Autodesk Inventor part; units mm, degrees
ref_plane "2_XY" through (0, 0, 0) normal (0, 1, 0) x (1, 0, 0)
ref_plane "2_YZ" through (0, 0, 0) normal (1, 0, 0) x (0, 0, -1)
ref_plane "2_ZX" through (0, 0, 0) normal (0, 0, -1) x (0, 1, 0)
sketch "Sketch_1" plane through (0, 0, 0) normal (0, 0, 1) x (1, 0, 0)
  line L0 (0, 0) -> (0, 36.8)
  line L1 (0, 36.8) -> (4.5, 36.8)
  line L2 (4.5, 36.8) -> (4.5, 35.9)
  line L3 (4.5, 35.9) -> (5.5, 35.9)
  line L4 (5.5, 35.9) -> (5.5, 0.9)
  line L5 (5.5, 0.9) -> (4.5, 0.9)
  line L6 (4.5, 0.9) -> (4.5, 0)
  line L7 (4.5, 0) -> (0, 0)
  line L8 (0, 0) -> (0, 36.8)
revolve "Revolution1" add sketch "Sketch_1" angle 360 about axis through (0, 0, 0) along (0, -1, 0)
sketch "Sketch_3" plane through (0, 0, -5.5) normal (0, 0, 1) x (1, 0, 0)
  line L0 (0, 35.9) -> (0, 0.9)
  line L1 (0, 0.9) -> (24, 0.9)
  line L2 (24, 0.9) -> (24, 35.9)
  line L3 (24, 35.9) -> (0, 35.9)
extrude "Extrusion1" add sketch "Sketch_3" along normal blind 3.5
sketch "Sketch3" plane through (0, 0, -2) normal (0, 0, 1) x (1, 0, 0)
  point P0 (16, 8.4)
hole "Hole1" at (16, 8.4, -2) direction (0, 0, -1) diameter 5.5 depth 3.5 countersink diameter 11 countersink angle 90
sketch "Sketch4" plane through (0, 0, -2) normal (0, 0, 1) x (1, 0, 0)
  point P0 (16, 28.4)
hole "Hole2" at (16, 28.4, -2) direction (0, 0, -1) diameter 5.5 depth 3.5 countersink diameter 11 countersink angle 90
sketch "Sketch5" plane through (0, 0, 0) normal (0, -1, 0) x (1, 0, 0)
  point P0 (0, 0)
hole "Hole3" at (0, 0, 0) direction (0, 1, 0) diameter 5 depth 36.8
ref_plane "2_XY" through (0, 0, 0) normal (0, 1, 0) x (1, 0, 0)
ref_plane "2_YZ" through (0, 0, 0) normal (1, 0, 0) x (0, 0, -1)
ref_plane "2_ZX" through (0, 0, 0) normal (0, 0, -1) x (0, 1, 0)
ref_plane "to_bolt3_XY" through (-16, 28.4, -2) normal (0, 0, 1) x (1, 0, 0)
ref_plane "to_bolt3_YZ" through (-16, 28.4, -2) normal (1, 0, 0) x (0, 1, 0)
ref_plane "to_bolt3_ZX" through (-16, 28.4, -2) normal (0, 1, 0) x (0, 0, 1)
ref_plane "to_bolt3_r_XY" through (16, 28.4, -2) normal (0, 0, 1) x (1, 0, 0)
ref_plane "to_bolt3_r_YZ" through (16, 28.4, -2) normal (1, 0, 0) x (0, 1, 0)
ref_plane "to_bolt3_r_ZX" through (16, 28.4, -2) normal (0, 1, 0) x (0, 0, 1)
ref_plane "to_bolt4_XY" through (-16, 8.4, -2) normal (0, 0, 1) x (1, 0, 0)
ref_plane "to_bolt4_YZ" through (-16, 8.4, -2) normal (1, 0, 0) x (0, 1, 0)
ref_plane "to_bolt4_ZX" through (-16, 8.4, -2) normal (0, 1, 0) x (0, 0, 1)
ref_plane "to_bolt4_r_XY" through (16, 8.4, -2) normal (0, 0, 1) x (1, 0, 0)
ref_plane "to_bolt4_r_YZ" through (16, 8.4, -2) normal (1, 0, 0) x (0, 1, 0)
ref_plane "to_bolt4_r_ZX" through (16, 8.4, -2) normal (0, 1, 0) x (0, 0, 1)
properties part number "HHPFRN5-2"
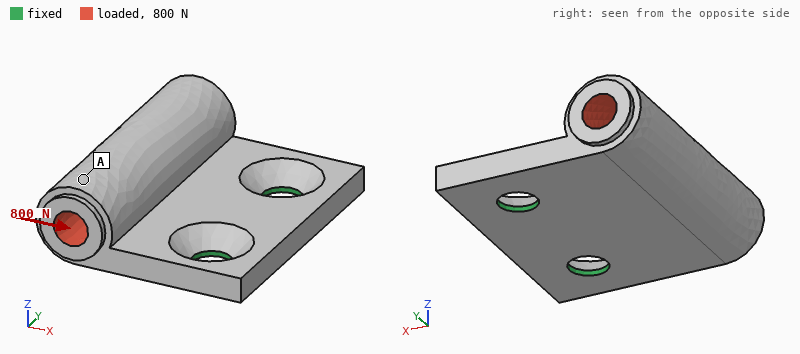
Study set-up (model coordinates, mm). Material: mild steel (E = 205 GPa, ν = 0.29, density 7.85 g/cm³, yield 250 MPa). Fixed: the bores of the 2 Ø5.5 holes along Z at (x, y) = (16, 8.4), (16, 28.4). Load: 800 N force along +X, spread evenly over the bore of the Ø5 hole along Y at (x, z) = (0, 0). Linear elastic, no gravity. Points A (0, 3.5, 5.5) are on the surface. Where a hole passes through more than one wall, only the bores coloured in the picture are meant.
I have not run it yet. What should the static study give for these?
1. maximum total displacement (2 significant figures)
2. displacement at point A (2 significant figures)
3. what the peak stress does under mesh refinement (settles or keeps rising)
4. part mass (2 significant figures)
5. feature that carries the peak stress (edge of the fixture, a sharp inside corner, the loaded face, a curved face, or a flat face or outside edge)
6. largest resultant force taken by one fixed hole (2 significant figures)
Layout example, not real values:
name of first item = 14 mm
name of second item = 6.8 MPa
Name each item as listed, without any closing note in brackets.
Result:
maximum total displacement = 51 µm
displacement at point A = 44 µm
what the peak stress does under mesh refinement = keeps rising
part mass = 38 g
feature that carries the peak stress = edge of the fixture
largest resultant force taken by one fixed hole = 400 N
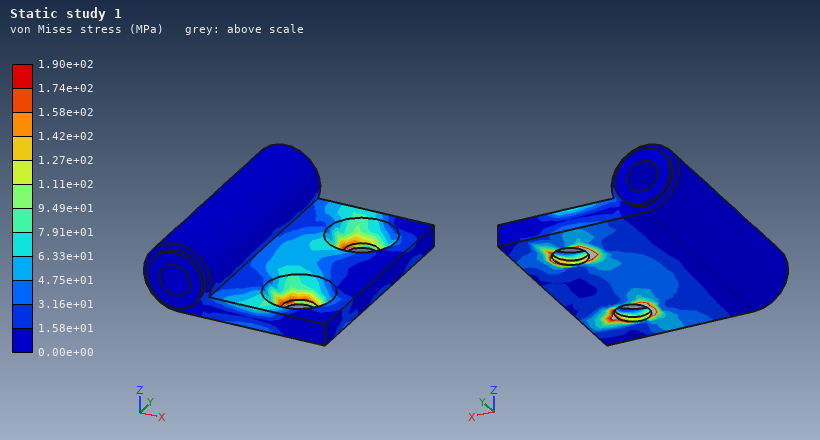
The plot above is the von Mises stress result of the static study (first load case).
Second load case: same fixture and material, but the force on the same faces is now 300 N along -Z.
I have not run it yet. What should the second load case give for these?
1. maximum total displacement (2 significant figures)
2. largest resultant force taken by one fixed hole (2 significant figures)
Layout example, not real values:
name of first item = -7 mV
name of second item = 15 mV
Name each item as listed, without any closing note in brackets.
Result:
maximum total displacement = 52 µm
largest resultant force taken by one fixed hole = 160 N
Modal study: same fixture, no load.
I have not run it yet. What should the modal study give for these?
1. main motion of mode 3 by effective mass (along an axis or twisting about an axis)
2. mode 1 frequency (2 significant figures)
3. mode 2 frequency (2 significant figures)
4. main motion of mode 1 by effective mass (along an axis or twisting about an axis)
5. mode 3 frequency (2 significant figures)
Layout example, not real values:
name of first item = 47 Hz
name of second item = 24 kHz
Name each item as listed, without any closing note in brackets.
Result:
main motion of mode 3 by effective mass = along Y
mode 1 frequency = 2800 Hz
mode 2 frequency = 8000 Hz
main motion of mode 1 by effective mass = along Z
mode 3 frequency = 16 kHz
